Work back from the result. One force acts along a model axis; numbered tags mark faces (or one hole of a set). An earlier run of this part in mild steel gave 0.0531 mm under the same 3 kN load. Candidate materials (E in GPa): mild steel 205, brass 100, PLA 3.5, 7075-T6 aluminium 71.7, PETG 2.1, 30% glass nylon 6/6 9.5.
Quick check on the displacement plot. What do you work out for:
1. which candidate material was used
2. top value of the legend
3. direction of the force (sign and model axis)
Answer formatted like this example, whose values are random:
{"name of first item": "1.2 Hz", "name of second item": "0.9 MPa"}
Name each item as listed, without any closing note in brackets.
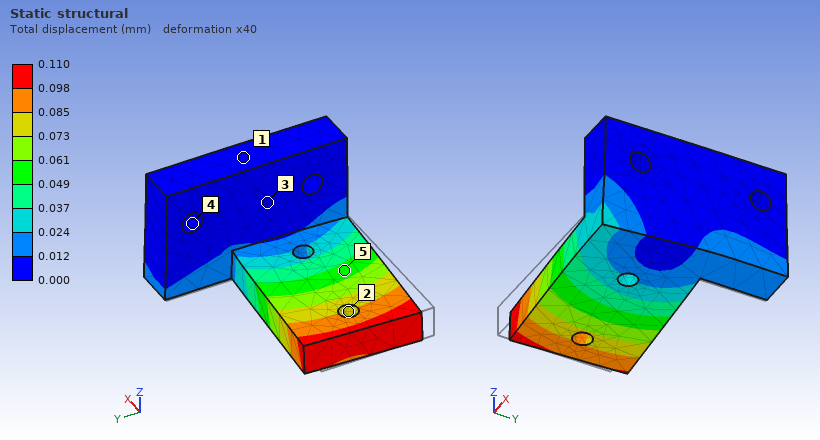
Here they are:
{"which candidate material was used": "brass", "top value of the legend": "0.110 mm", "direction of the force": "+Y"}
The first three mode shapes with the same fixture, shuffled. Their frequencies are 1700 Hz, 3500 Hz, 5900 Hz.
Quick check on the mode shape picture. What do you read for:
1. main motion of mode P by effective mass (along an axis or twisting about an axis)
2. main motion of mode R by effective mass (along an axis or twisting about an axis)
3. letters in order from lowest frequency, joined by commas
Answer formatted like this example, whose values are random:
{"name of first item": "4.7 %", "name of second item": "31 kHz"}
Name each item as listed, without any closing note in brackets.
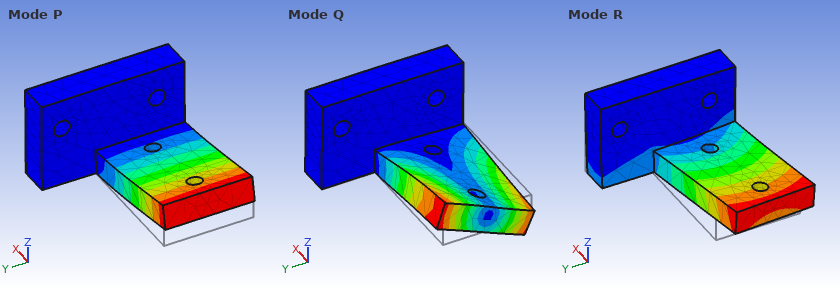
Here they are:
{"main motion of mode P by effective mass": "along Z", "main motion of mode R by effective mass": "along Y", "letters in order from lowest frequency, joined by commas": "P, R, Q"}
